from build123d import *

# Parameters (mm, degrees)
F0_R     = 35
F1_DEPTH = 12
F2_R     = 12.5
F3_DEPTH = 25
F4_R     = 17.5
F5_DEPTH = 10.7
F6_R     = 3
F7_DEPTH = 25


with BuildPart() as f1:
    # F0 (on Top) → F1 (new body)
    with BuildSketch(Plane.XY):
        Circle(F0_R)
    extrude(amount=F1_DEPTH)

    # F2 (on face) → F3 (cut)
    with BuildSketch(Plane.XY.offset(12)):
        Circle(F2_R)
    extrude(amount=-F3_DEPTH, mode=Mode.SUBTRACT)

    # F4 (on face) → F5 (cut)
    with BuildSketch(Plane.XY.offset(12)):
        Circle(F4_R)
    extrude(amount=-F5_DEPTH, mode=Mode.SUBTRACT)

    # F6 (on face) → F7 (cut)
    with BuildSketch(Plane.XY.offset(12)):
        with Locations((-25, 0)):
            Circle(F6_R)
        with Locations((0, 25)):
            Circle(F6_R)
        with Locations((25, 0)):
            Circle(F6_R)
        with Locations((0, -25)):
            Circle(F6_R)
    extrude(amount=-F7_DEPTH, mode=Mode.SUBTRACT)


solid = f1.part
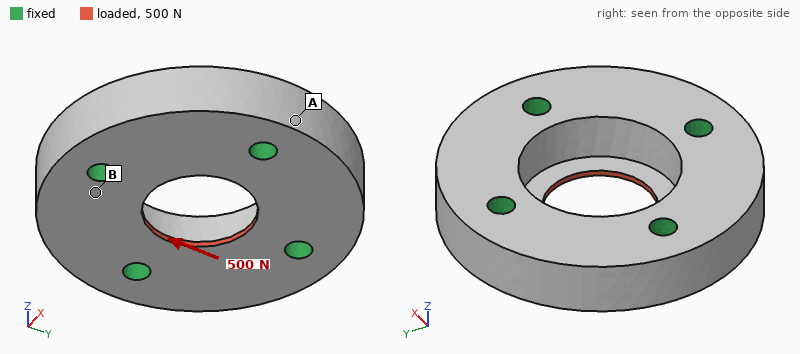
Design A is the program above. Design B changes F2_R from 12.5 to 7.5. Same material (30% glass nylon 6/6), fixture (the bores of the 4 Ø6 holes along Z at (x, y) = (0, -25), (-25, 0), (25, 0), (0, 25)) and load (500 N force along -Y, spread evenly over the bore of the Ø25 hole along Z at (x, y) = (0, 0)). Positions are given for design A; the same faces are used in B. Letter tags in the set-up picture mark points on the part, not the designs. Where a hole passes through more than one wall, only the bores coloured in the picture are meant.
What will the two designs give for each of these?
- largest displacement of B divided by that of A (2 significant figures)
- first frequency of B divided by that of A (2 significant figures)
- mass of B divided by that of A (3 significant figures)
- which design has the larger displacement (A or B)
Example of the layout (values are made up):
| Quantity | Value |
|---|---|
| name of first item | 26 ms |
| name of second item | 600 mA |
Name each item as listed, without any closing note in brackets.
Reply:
| Quantity | Value |
|---|---|
| largest displacement of B divided by that of A | 1.6 |
| first frequency of B divided by that of A | 0.64 |
| mass of B divided by that of A | 1.01 |
| which design has the larger displacement | B |
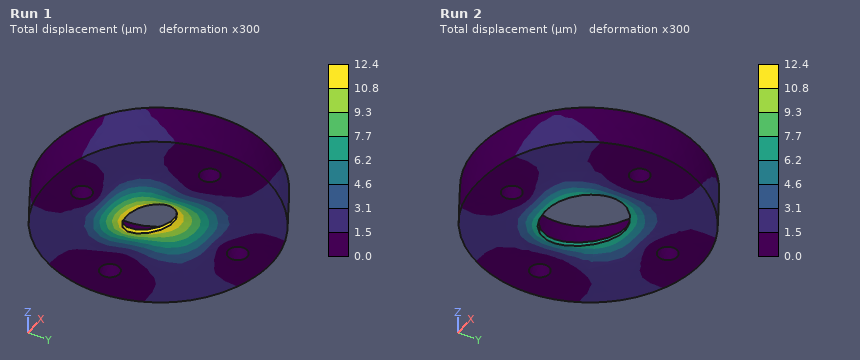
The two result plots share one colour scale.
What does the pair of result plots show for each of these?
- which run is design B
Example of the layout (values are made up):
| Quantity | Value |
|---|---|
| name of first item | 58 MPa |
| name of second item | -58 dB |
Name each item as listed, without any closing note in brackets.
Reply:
| Quantity | Value |
|---|---|
| which run is design B | Run 1 |
